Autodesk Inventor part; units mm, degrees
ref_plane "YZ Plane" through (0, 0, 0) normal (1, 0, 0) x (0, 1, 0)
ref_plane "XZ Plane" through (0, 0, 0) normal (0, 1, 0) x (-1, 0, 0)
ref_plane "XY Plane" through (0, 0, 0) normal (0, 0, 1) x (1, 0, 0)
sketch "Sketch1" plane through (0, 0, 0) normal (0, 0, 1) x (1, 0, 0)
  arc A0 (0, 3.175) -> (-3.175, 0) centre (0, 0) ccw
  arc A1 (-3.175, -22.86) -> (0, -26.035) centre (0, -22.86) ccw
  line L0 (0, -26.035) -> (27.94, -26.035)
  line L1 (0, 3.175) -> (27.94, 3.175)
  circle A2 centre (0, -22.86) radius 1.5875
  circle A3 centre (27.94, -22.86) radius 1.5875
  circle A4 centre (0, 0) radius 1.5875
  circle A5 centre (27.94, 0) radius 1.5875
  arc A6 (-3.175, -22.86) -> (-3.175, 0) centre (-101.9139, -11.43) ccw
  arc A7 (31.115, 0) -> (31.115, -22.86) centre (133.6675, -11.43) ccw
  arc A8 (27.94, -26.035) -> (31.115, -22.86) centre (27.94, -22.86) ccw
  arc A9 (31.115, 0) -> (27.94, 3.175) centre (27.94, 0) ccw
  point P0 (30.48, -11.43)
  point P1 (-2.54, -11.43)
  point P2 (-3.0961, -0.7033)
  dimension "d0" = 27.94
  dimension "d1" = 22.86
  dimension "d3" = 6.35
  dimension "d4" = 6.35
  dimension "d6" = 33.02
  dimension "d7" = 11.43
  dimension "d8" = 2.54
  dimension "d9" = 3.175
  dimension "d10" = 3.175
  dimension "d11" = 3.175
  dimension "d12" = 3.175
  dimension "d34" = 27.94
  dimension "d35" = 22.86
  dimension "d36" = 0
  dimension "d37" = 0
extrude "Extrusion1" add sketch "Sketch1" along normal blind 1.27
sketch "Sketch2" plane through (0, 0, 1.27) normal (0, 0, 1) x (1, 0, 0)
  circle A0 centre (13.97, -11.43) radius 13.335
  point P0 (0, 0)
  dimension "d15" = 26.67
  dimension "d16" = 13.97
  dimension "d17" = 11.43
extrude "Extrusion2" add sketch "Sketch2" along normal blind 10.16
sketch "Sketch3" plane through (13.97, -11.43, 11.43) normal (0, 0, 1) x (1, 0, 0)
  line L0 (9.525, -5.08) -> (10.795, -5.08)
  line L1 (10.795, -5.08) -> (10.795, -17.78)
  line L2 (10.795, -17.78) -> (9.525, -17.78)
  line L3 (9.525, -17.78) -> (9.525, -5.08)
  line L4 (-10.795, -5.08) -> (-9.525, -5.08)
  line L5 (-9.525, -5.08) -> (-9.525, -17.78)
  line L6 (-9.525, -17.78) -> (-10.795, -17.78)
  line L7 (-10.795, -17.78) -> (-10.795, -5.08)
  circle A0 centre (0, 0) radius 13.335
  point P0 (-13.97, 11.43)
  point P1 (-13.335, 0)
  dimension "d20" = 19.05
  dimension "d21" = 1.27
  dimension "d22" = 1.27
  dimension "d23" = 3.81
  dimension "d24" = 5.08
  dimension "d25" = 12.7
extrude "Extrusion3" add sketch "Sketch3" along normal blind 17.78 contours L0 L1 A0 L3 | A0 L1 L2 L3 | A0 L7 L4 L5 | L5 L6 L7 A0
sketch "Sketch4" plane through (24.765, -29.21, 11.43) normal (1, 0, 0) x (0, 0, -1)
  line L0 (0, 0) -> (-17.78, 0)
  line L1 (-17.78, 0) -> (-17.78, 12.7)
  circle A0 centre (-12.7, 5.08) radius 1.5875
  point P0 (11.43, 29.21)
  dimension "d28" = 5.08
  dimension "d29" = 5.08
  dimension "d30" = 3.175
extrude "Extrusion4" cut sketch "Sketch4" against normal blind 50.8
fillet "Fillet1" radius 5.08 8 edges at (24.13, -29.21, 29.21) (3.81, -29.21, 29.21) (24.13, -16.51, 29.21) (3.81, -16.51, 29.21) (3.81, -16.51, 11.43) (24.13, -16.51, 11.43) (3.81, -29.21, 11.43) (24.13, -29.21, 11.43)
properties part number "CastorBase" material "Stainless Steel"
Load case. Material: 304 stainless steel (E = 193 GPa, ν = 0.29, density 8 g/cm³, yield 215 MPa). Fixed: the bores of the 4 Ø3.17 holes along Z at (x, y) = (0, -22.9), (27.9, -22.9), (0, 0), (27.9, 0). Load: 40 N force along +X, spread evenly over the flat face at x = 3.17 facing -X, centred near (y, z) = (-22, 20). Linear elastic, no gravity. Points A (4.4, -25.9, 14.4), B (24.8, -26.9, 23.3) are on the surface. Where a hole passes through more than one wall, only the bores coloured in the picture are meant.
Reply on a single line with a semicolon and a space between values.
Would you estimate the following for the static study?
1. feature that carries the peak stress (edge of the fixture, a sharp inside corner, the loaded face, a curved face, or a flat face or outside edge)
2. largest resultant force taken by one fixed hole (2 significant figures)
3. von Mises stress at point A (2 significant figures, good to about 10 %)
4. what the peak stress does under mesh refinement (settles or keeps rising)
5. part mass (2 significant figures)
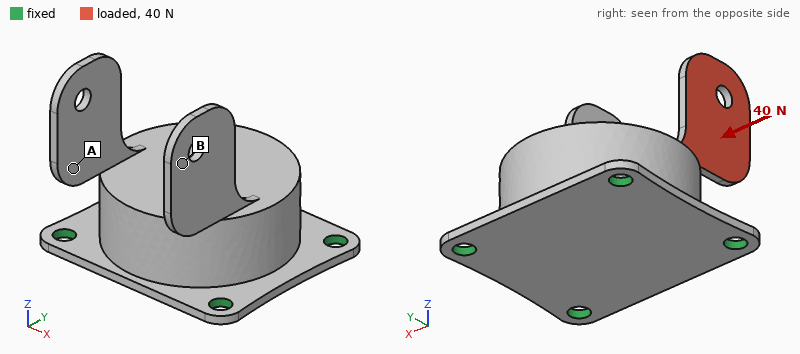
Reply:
a sharp inside corner; 23 N; 30 MPa; keeps rising; 59 g
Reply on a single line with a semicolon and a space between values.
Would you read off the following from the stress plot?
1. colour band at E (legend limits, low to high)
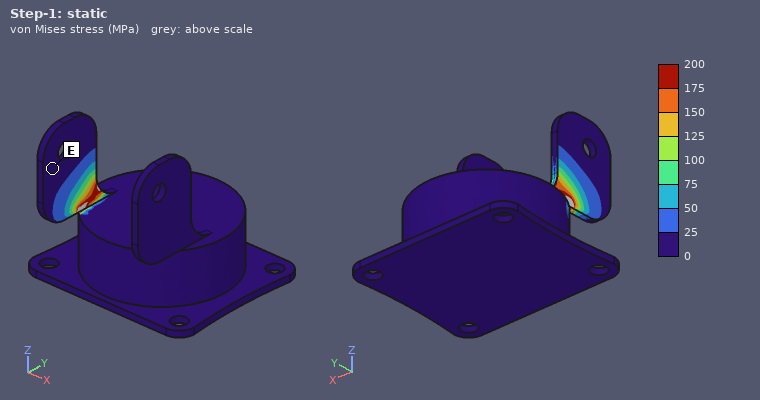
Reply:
0 to 25 MPa
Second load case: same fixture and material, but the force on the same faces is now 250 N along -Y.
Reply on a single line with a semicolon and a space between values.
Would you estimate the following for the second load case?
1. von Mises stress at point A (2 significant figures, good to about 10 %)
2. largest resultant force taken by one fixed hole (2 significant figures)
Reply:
23 MPa; 150 N
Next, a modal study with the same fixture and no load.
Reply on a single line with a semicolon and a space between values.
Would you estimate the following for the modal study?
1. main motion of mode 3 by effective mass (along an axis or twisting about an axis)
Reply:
along Y
